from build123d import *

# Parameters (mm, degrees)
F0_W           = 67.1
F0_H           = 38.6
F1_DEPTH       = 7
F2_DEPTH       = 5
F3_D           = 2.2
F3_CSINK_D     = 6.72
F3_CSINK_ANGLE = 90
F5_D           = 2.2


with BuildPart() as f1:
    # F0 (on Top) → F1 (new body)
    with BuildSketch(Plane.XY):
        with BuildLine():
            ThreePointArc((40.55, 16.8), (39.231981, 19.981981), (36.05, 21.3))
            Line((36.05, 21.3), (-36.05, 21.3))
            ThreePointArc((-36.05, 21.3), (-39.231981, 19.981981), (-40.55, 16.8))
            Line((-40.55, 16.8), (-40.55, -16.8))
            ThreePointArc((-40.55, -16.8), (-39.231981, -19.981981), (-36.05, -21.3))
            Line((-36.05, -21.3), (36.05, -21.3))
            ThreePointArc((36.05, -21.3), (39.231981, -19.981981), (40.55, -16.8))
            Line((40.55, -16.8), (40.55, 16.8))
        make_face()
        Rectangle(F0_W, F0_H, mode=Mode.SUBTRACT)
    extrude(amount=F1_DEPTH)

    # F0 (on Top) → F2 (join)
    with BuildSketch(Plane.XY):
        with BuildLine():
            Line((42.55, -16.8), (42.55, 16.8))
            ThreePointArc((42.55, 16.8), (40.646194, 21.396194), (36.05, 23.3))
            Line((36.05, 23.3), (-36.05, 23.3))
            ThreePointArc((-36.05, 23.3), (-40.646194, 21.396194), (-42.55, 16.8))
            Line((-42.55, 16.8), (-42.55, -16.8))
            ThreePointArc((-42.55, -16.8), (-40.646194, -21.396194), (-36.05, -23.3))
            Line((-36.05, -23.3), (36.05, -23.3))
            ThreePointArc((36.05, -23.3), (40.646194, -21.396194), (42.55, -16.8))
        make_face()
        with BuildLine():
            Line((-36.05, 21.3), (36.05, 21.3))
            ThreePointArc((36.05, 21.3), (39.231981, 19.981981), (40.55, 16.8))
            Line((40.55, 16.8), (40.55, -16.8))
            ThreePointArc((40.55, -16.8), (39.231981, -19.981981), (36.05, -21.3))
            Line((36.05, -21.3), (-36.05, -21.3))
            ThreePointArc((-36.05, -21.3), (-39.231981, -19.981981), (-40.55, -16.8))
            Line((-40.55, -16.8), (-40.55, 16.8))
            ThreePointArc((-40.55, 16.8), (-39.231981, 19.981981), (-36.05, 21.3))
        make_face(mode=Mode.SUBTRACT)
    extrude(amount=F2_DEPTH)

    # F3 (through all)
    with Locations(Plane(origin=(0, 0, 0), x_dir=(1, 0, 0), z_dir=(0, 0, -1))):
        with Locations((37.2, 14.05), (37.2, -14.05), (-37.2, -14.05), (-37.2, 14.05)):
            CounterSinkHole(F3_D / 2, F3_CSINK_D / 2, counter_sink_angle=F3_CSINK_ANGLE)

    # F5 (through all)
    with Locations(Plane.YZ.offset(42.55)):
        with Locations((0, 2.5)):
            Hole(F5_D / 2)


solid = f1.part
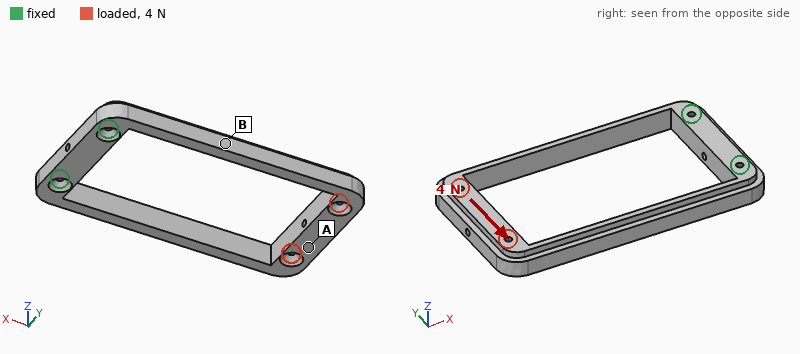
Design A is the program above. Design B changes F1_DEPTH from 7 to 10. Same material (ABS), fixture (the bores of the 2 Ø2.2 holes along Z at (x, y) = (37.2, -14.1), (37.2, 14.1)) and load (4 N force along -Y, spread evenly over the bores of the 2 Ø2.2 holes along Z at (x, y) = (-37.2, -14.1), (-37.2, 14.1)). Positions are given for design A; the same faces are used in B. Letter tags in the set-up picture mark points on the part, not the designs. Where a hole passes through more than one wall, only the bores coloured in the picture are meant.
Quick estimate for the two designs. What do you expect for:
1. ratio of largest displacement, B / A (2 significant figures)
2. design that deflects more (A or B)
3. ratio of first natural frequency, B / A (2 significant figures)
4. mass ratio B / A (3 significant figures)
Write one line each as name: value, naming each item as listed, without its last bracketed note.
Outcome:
ratio of largest displacement, B / A: 0.91
design that deflects more: A
ratio of first natural frequency, B / A: 1.1
mass ratio B / A: 1.31
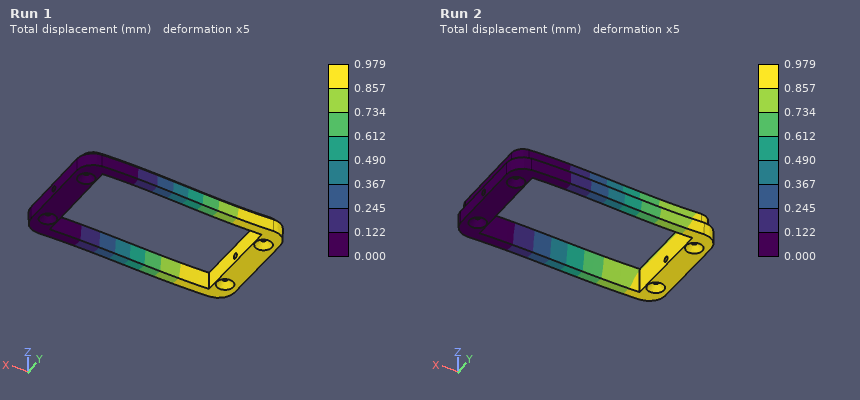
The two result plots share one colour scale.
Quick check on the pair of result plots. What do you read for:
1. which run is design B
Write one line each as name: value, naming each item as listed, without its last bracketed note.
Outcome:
which run is design B: Run 2
